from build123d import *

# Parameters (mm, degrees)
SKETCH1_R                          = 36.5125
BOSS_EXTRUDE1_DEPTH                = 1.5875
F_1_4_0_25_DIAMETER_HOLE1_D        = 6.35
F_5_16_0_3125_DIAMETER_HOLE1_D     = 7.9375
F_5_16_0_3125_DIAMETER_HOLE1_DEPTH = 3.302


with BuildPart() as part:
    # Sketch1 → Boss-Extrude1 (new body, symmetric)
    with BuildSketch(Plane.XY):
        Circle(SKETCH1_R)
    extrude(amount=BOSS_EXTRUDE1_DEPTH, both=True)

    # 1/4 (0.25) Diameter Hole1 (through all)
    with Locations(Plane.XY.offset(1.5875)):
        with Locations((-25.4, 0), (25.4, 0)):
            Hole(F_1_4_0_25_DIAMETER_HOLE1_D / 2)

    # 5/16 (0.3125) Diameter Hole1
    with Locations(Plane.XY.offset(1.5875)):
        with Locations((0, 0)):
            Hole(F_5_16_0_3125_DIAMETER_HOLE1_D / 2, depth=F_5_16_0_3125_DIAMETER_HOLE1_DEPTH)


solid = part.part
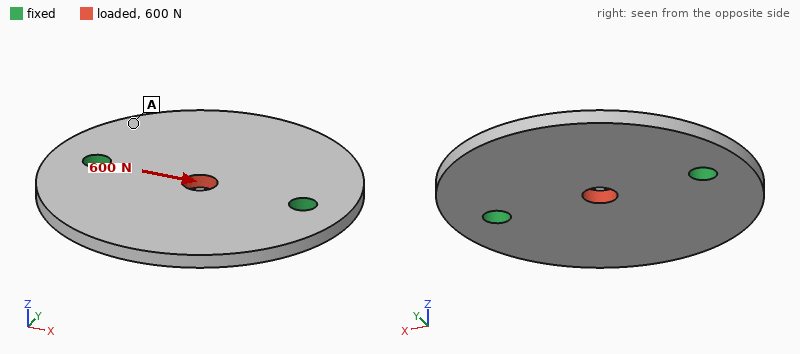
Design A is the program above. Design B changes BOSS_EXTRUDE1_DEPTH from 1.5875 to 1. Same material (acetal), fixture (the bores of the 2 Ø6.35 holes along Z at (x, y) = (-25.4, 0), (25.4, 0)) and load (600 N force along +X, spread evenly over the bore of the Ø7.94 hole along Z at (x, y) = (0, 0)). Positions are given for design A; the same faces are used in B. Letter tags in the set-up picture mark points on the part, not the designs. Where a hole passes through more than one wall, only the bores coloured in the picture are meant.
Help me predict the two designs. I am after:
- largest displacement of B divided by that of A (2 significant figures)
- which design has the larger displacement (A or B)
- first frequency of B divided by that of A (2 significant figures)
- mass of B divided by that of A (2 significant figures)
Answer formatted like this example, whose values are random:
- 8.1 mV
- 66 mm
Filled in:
- 1.6
- B
- 0.65
- 0.63
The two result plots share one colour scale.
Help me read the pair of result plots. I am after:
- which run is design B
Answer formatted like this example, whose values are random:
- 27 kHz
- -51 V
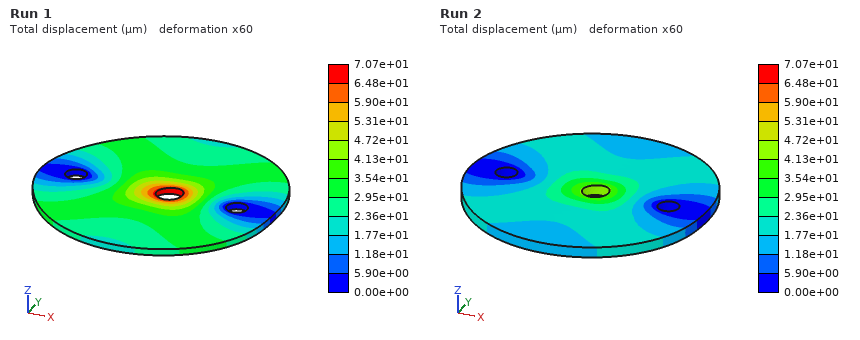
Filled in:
- Run 1
